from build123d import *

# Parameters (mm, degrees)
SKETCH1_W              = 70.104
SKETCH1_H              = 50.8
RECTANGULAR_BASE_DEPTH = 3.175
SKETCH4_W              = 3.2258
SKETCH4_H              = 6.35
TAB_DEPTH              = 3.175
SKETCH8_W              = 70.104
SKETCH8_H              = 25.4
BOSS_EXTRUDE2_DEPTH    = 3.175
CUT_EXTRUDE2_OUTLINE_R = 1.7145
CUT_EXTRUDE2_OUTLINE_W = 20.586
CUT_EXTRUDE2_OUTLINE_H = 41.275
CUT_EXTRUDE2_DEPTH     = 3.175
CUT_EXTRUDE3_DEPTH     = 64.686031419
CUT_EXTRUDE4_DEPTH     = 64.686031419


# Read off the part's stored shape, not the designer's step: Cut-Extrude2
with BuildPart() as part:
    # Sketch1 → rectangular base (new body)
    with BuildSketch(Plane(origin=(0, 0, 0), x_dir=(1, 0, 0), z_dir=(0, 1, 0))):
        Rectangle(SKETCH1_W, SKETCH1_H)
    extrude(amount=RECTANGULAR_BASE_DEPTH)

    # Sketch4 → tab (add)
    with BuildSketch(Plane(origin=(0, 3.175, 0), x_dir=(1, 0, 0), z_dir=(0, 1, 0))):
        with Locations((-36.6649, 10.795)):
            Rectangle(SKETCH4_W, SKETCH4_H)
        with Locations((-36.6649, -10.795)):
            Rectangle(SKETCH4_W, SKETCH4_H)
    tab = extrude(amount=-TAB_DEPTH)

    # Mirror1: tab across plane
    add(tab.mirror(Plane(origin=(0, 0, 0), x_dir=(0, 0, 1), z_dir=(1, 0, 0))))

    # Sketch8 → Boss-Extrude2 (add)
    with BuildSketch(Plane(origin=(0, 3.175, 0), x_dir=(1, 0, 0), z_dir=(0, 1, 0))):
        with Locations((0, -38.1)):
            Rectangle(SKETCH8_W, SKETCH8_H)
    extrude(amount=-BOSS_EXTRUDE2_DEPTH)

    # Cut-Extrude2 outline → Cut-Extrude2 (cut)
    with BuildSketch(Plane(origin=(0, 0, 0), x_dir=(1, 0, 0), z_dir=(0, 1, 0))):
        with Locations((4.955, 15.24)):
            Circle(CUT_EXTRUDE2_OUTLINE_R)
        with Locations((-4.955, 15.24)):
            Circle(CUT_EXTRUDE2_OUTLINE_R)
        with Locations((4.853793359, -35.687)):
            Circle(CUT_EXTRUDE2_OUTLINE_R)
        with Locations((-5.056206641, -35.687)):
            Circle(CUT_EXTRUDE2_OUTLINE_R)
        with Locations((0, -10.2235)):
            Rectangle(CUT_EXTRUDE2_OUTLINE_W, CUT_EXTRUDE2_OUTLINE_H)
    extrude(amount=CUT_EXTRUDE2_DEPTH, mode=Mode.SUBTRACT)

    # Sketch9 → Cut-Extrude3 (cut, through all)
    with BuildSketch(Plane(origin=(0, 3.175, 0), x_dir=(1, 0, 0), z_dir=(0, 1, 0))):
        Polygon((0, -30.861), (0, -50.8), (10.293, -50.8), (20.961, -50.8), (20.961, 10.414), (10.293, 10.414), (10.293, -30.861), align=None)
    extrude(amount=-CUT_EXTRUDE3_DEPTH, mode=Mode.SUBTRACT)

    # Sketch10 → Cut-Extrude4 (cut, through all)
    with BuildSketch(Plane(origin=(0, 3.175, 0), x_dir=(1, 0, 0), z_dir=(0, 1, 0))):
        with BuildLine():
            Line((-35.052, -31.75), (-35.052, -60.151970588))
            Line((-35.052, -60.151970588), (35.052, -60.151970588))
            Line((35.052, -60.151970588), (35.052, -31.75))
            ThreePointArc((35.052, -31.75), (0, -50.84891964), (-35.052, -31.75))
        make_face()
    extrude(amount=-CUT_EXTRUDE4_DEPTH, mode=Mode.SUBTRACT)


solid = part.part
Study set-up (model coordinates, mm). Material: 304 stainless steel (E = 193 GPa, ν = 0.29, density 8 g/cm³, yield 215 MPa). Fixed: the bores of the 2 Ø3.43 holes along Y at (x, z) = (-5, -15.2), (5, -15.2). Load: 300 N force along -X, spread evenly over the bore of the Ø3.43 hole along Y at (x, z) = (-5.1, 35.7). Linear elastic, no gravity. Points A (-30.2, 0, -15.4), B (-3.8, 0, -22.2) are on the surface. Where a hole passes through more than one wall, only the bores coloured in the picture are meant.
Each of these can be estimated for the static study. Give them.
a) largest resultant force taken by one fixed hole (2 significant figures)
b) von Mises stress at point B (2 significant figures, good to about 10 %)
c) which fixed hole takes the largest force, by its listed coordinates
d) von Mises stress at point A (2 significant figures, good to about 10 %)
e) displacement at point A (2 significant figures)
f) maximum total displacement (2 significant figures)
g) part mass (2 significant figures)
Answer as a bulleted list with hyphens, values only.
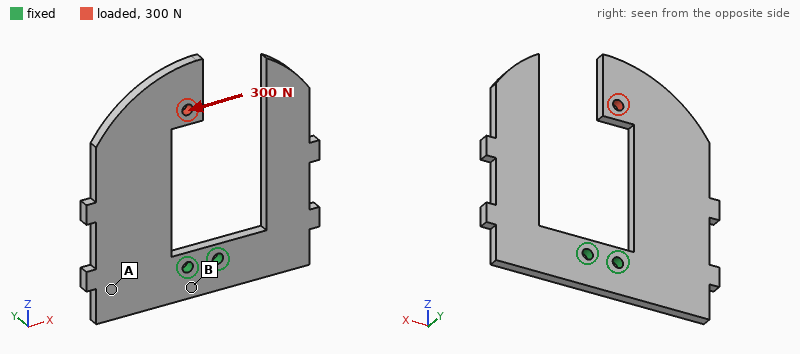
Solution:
- 1.2 kN
- 67 MPa
- (-5, -15.2)
- 22 MPa
- 0.037 mm
- 0.14 mm
- 85 g
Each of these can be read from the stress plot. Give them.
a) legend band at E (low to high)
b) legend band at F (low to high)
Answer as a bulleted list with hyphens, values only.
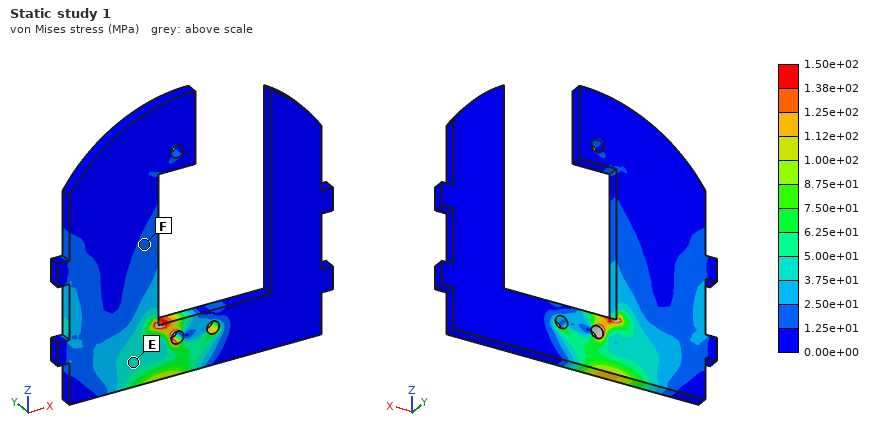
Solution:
- 3.75e+01 to 5.00e+01 MPa
- 1.25e+01 to 2.50e+01 MPa
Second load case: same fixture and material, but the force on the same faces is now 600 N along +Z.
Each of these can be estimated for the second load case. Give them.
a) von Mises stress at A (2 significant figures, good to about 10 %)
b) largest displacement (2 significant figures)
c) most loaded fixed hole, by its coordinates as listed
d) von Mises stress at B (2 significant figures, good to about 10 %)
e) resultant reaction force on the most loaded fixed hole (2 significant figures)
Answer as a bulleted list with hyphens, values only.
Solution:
- 11 MPa
- 51 µm
- (-5, -15.2)
- 6.1 MPa
- 570 N
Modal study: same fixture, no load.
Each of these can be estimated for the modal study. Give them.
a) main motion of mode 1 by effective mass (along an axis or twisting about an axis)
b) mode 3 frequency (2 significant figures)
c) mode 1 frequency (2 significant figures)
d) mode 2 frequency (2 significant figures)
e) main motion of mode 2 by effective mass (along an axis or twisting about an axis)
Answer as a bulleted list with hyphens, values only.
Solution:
- along Y
- 1300 Hz
- 440 Hz
- 560 Hz
- along Y
